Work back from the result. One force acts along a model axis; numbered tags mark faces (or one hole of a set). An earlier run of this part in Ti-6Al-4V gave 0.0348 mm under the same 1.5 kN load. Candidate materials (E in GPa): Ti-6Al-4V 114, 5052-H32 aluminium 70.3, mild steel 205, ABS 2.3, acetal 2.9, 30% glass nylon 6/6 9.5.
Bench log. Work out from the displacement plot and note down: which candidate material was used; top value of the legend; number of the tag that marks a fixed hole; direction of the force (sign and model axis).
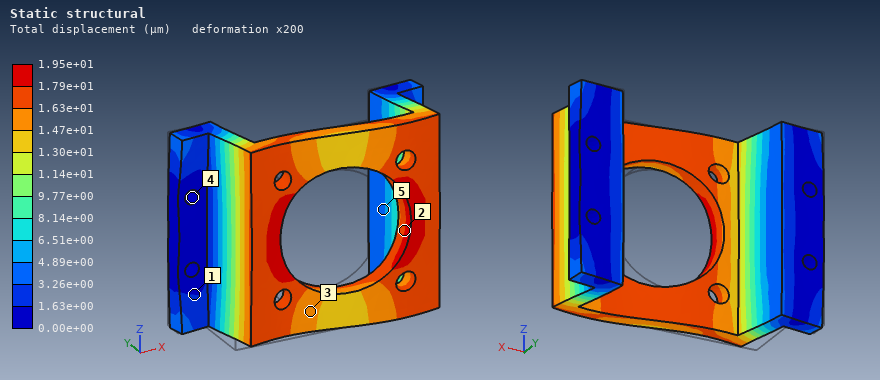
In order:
mild steel
1.95e+01 µm
4
+X
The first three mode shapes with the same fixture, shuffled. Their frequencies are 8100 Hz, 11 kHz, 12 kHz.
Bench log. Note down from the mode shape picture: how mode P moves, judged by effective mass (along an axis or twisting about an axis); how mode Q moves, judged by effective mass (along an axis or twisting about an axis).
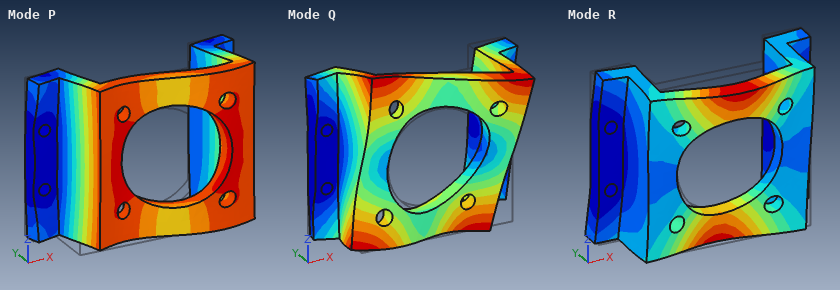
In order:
along X
twisting about Y
